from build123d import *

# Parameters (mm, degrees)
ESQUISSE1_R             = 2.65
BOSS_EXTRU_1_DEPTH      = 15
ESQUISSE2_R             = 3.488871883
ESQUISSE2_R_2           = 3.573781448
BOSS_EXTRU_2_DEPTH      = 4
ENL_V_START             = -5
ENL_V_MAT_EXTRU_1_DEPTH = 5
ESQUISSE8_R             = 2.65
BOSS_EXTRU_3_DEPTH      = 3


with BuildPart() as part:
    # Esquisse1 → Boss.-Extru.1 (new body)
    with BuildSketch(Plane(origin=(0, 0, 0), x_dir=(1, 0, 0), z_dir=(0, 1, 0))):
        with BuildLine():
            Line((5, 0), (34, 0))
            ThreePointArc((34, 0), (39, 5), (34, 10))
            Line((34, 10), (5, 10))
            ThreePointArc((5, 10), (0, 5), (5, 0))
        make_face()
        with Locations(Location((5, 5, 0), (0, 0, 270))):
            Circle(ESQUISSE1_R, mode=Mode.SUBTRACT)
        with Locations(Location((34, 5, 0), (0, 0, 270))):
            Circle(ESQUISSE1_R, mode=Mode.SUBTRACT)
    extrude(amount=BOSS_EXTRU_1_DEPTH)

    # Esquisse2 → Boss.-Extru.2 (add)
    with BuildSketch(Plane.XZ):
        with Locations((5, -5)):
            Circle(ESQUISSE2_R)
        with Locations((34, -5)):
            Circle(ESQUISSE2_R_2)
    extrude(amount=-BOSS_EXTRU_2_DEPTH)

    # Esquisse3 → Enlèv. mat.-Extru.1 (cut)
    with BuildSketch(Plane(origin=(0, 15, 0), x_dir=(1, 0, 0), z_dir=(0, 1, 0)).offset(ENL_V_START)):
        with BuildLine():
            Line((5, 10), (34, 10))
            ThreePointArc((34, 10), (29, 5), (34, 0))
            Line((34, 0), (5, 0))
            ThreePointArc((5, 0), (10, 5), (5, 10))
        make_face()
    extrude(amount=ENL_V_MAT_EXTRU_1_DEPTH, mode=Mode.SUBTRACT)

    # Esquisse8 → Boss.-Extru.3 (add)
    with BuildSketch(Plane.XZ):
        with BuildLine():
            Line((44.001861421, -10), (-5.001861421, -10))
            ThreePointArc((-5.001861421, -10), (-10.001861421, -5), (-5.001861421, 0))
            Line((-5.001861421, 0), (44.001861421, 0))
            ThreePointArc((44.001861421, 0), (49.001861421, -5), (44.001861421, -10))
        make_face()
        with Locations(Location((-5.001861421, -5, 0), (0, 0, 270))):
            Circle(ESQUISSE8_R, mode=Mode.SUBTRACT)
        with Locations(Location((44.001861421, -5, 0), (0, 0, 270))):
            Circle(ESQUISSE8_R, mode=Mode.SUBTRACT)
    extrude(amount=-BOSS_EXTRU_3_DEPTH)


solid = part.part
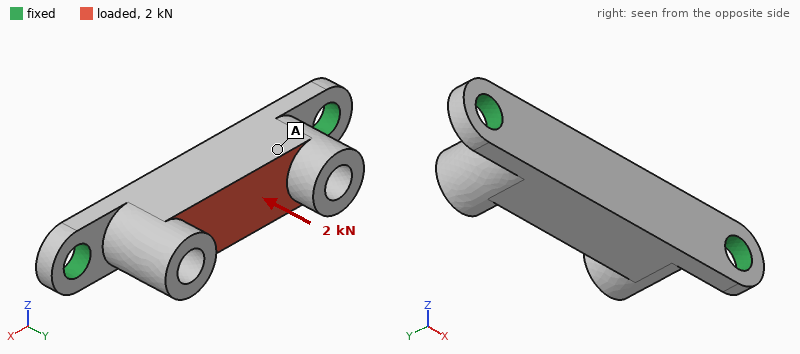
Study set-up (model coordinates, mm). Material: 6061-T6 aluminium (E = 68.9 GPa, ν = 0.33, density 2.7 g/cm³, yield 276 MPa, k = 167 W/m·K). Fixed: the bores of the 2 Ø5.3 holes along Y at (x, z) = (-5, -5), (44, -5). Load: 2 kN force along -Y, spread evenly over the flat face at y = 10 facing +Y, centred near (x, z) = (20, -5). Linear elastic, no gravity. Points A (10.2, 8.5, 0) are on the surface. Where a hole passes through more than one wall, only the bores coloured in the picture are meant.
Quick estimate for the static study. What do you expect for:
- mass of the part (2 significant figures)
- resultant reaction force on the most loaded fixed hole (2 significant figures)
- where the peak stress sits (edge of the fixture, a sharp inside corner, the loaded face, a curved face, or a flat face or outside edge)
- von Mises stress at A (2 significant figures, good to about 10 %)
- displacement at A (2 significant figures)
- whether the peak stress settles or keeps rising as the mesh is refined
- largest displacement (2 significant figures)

12 g
1.6 kN
edge of the fixture
43 MPa
39 µm
keeps rising
48 µm
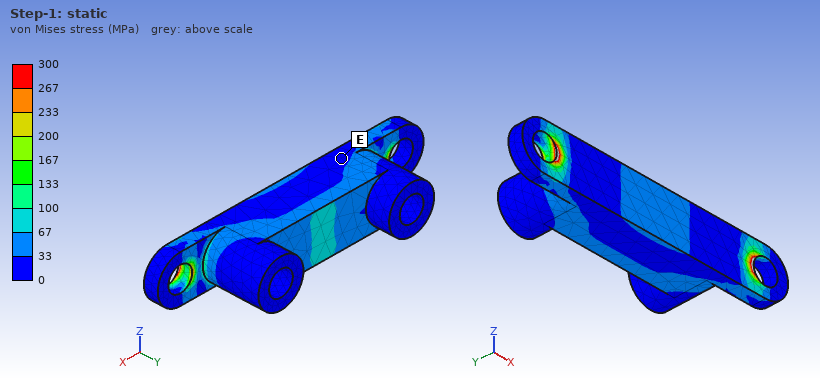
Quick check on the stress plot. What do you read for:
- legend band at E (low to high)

0 to 33 MPa
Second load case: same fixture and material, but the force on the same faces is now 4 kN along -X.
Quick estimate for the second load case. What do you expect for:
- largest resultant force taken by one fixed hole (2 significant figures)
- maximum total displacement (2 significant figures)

2.2 kN
19 µm
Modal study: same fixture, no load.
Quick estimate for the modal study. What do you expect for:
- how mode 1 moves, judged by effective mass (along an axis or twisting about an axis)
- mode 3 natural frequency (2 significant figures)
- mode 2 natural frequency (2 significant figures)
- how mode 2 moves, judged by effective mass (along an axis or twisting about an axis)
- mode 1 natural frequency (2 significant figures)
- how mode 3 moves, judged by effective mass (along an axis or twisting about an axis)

along Z
16 kHz
12 kHz
along Y
7100 Hz
along Z
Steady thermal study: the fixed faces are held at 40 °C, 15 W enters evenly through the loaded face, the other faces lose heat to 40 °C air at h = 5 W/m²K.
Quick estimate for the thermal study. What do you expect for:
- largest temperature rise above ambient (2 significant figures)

16 K
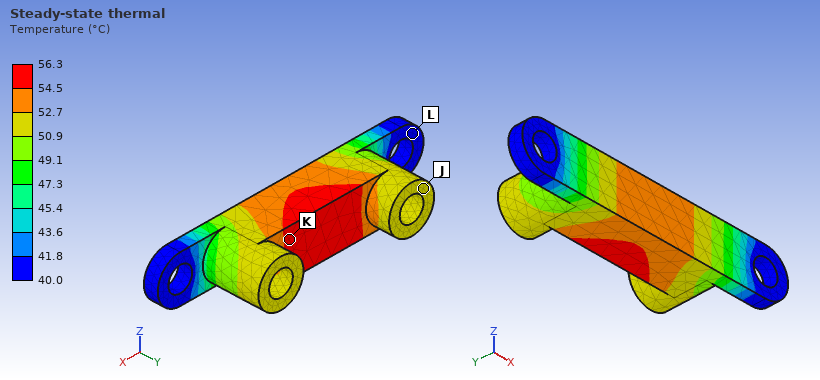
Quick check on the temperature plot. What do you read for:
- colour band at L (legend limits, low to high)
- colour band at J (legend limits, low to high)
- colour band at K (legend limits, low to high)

40.0 to 41.8 °C
50.9 to 52.7 °C
54.5 to 56.3 °C
